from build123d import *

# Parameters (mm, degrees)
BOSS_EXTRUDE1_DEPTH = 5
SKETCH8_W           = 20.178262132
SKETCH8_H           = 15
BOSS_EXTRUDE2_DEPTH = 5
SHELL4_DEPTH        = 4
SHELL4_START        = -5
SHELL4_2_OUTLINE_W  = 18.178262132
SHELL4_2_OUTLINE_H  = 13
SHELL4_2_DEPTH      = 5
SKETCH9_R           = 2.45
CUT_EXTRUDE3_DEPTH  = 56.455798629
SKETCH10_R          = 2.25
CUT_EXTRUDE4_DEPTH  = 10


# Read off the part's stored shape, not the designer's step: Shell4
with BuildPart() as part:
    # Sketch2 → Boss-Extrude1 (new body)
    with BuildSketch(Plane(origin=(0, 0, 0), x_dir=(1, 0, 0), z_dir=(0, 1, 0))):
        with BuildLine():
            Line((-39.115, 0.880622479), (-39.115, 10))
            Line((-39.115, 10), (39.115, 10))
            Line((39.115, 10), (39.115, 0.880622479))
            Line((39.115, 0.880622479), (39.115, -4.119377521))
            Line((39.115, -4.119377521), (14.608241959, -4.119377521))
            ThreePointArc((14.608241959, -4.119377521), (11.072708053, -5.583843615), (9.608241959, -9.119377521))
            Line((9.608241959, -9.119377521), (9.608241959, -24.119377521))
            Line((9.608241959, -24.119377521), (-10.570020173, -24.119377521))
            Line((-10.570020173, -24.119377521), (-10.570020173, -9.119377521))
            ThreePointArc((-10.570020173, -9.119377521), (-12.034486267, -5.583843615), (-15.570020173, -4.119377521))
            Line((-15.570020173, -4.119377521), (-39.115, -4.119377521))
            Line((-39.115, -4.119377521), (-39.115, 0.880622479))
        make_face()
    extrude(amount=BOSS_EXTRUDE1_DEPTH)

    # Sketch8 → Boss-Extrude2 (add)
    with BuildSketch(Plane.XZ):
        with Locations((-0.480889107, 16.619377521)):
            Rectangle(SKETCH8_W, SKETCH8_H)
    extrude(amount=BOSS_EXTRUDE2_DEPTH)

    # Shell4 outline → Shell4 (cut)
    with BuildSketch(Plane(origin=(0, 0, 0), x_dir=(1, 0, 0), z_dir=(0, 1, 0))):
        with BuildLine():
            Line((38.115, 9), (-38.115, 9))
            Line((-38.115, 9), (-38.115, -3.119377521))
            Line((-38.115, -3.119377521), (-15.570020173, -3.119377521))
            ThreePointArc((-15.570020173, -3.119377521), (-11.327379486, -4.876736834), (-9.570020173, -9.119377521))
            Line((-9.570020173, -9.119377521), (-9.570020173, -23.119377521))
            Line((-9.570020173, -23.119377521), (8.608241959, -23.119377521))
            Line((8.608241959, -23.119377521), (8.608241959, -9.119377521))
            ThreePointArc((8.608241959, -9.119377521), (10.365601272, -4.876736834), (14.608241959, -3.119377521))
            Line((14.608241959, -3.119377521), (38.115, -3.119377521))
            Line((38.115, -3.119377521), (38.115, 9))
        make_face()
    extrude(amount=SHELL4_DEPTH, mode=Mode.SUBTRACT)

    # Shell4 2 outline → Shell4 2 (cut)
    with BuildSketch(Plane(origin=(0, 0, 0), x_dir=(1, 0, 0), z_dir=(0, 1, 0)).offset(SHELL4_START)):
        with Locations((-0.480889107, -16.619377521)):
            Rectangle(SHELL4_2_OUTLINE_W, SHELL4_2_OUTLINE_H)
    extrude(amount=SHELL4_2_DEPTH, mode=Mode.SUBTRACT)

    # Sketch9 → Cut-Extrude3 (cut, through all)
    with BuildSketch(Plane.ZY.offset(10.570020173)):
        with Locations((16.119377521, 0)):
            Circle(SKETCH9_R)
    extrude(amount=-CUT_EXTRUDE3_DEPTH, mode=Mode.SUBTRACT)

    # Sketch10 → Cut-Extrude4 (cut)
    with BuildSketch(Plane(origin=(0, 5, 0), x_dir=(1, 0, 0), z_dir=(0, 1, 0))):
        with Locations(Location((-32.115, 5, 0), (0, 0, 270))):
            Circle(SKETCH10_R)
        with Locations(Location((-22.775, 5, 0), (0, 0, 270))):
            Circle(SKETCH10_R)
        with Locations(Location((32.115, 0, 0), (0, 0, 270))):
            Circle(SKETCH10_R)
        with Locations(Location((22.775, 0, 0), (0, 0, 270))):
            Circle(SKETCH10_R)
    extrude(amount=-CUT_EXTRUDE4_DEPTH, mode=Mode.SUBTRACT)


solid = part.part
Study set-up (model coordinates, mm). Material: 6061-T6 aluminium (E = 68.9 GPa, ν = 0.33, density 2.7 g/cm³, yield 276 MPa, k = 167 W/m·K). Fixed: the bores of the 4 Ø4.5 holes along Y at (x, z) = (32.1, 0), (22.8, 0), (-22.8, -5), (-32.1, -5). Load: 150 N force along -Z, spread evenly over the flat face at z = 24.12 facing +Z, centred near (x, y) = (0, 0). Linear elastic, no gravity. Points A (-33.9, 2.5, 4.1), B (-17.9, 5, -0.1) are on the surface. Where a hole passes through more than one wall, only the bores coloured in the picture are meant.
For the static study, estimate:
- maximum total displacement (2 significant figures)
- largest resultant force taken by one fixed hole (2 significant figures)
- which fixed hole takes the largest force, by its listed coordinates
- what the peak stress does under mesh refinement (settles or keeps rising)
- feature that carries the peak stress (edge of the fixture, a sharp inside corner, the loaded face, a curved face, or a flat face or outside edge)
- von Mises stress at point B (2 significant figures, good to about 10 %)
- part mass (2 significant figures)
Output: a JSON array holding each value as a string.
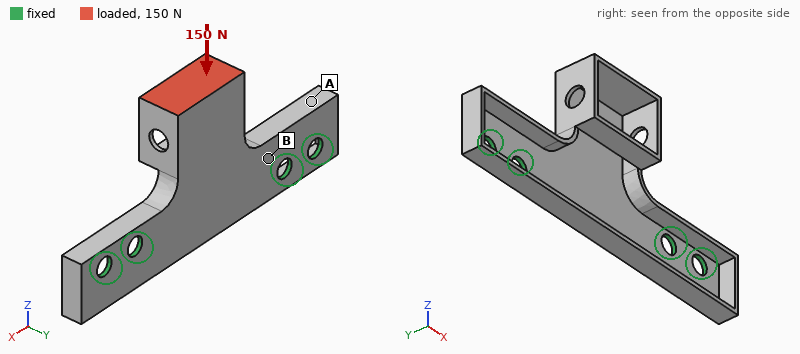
["0.68 mm", "120 N", "(-22.8, -5)", "keeps rising", "edge of the fixture", "48 MPa", "7.1 g"]
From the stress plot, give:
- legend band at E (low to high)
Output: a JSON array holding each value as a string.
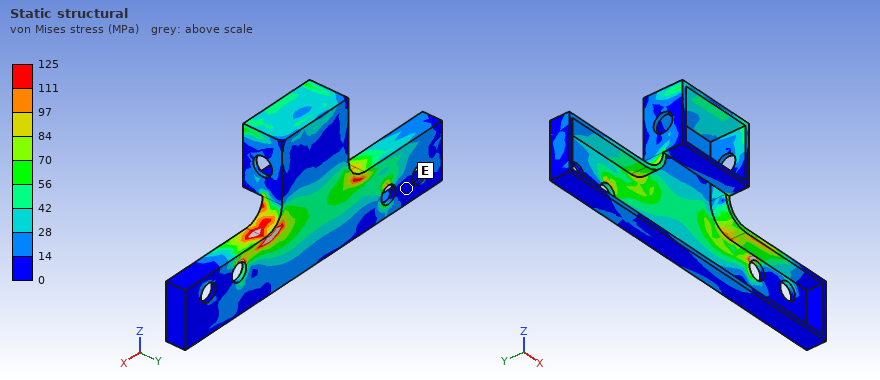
["0 to 14 MPa"]
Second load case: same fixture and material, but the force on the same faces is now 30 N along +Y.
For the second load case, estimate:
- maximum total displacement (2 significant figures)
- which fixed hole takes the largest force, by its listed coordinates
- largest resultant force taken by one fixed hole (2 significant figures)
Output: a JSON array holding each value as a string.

["0.70 mm", "(32.1, 0)", "110 N"]
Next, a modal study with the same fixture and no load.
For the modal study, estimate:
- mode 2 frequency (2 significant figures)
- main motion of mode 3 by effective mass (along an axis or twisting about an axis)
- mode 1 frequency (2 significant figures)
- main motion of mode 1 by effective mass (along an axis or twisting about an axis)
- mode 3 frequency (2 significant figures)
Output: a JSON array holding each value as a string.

["3100 Hz", "along Y", "970 Hz", "along Y", "5400 Hz"]
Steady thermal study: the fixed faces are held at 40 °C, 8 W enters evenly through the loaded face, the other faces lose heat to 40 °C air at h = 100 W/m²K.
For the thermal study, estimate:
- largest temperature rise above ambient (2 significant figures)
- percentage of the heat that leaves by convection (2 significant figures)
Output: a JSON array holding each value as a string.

["36 K", "58 %"]
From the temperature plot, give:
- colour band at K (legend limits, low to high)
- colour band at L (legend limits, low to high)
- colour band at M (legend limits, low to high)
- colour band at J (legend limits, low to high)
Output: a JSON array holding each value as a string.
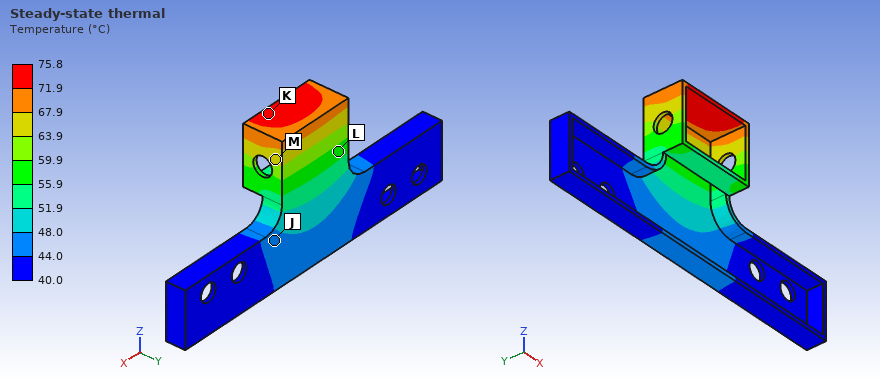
["71.9 to 75.8 °C", "55.9 to 59.9 °C", "63.9 to 67.9 °C", "44.0 to 48.0 °C"]
